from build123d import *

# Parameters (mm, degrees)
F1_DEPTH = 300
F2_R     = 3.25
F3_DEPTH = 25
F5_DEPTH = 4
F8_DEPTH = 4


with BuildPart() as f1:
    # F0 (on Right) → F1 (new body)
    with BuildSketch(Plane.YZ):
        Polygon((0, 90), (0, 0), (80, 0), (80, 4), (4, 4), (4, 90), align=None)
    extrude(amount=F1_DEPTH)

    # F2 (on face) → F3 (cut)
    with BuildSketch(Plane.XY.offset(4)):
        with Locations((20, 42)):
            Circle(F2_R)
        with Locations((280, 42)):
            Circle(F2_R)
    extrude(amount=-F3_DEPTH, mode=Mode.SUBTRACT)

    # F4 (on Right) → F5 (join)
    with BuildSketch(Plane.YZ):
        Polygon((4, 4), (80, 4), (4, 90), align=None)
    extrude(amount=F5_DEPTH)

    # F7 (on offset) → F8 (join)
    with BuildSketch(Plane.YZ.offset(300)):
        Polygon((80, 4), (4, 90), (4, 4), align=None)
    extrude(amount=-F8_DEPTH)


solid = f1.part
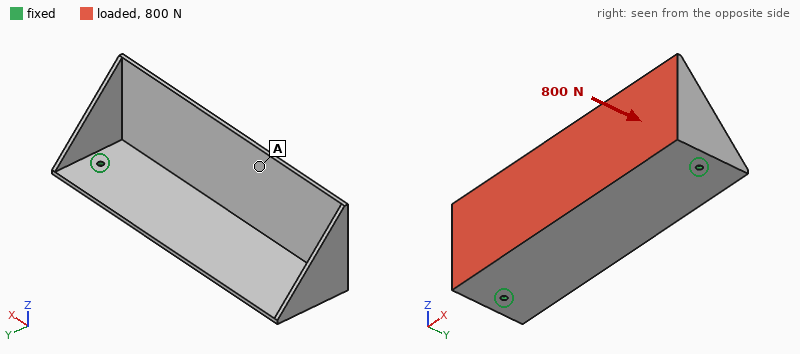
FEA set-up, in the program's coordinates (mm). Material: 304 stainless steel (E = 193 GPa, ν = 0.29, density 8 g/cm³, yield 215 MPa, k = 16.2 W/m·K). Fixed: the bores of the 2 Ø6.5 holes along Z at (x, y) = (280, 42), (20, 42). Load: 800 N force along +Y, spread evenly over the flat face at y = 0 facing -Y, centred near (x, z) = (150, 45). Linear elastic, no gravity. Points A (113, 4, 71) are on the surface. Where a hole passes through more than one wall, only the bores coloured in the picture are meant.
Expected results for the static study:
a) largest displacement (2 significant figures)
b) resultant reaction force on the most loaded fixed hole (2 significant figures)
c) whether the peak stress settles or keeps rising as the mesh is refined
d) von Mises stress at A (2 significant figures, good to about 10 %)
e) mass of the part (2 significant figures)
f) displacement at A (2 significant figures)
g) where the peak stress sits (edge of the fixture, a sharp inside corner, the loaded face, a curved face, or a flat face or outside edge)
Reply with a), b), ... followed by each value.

a) 0.50 mm
b) 430 N
c) keeps rising
d) 12 MPa
e) 1.8 kg
f) 0.38 mm
g) edge of the fixture
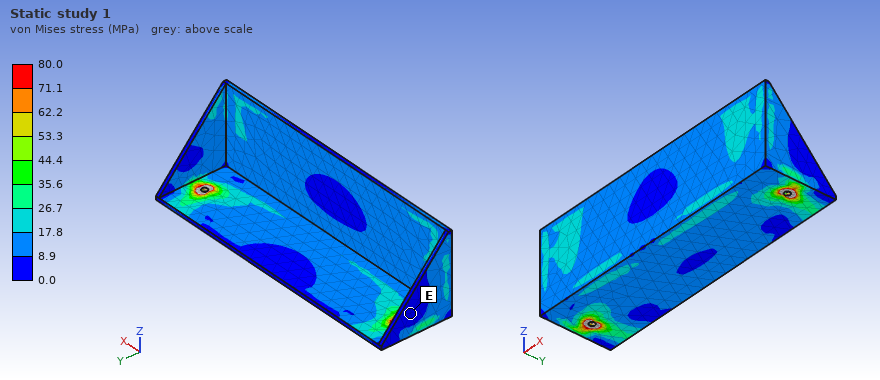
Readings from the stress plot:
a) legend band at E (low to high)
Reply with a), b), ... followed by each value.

a) 0.0 to 8.9 MPa
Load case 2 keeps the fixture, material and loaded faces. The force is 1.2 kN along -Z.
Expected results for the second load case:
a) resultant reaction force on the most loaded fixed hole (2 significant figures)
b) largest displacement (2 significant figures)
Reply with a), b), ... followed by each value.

a) 600 N
b) 0.35 mm
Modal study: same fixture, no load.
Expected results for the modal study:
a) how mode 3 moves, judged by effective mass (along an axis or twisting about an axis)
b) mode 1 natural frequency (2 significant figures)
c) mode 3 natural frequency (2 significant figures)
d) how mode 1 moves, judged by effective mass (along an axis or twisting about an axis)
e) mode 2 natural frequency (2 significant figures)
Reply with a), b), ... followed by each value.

a) along Z
b) 260 Hz
c) 460 Hz
d) along Y
e) 430 Hz
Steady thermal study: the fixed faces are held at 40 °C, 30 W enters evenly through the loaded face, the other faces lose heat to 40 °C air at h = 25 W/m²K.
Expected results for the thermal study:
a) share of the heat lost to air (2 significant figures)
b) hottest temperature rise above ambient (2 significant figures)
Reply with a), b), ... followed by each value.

a) 94 %
b) 32 K
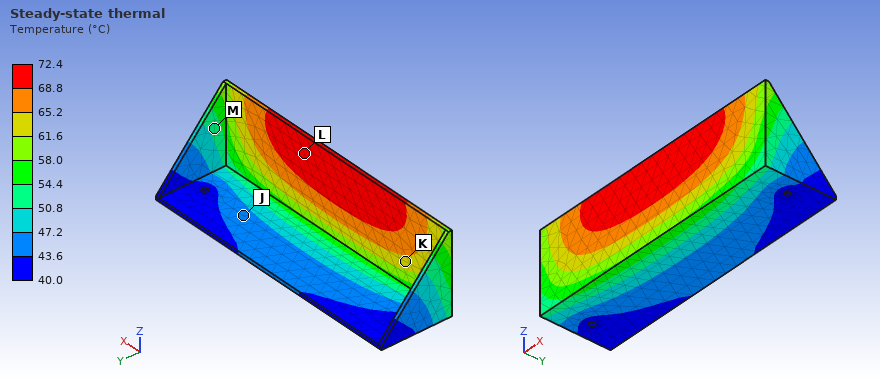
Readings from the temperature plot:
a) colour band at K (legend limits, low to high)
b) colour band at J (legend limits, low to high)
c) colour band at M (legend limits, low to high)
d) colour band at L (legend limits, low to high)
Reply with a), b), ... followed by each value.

a) 61.6 to 65.2 °C
b) 43.6 to 47.2 °C
c) 50.8 to 54.4 °C
d) 68.8 to 72.4 °C
